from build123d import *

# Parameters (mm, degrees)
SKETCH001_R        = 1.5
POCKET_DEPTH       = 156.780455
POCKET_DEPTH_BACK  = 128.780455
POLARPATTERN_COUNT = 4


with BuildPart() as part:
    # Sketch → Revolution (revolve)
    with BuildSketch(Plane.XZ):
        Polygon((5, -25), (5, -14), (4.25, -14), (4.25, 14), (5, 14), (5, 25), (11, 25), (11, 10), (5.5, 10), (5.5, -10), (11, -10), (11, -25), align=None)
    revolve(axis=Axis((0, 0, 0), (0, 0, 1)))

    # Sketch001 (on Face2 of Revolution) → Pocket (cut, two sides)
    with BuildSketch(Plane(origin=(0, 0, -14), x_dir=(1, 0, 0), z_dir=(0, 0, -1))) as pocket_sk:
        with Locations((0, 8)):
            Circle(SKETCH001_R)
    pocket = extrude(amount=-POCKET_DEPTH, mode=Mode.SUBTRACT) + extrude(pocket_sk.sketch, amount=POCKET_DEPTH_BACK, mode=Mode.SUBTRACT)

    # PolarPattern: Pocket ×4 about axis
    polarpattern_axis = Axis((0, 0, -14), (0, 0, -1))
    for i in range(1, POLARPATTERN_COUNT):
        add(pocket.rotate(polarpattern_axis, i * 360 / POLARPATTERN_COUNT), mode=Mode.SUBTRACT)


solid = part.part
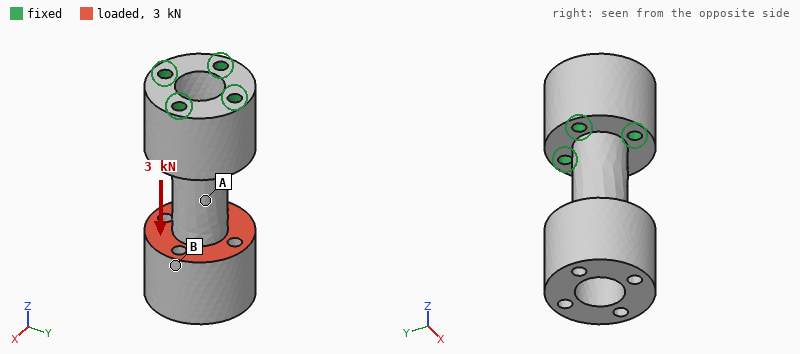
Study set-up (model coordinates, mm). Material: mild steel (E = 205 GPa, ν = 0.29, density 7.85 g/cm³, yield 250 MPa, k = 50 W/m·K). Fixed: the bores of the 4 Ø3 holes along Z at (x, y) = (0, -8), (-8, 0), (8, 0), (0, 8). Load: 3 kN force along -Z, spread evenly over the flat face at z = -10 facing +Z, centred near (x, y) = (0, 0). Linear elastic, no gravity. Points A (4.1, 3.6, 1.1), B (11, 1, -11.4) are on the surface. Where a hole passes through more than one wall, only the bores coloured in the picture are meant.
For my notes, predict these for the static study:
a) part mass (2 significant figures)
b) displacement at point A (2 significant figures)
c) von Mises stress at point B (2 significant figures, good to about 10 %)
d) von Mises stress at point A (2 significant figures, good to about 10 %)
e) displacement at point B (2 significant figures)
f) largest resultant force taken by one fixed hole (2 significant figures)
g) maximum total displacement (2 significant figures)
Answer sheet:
72 g
4.3 µm
12 MPa
78 MPa
9.9 µm
790 N
10 µm
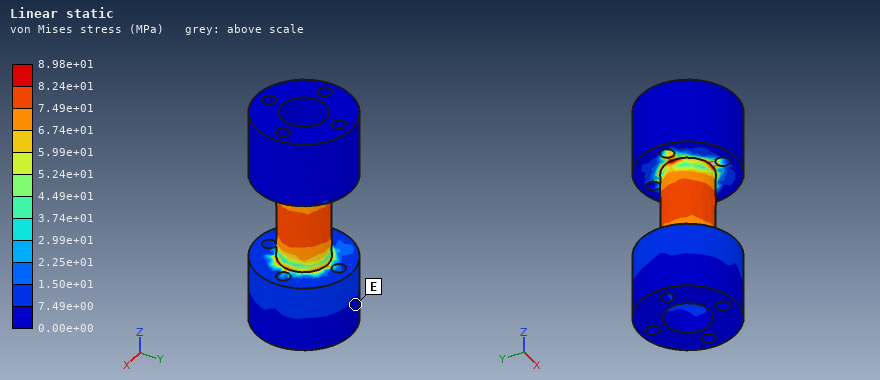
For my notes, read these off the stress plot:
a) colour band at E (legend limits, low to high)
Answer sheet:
0.00e+00 to 7.49e+00 MPa
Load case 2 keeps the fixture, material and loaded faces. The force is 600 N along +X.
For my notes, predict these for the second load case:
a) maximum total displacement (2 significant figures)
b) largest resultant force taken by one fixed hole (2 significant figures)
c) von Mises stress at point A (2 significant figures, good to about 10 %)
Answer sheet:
54 µm
970 N
67 MPa
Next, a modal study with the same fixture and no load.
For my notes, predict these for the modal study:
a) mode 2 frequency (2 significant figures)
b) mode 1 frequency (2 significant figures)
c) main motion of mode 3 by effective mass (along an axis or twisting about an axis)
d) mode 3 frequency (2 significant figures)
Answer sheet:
2600 Hz
2600 Hz
twisting about Z
5900 Hz
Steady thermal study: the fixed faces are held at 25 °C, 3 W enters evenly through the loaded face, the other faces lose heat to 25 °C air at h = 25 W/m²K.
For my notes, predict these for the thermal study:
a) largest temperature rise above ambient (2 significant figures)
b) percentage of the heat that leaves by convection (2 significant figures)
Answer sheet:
20 K
48 %
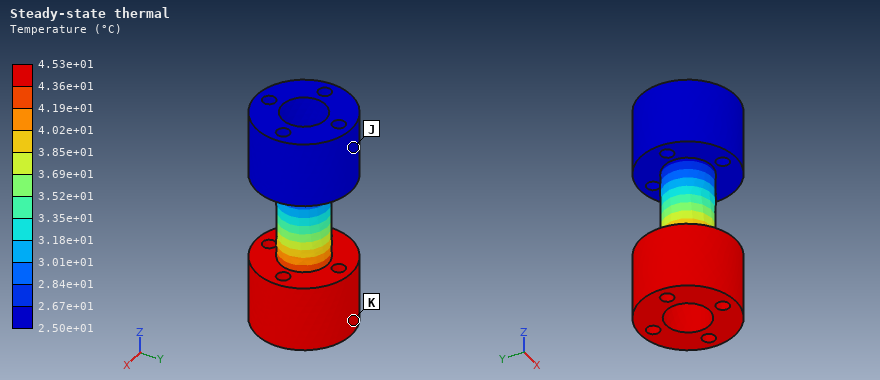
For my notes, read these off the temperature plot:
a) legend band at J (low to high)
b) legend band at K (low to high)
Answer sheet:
2.50e+01 to 2.67e+01 °C
4.36e+01 to 4.53e+01 °C
